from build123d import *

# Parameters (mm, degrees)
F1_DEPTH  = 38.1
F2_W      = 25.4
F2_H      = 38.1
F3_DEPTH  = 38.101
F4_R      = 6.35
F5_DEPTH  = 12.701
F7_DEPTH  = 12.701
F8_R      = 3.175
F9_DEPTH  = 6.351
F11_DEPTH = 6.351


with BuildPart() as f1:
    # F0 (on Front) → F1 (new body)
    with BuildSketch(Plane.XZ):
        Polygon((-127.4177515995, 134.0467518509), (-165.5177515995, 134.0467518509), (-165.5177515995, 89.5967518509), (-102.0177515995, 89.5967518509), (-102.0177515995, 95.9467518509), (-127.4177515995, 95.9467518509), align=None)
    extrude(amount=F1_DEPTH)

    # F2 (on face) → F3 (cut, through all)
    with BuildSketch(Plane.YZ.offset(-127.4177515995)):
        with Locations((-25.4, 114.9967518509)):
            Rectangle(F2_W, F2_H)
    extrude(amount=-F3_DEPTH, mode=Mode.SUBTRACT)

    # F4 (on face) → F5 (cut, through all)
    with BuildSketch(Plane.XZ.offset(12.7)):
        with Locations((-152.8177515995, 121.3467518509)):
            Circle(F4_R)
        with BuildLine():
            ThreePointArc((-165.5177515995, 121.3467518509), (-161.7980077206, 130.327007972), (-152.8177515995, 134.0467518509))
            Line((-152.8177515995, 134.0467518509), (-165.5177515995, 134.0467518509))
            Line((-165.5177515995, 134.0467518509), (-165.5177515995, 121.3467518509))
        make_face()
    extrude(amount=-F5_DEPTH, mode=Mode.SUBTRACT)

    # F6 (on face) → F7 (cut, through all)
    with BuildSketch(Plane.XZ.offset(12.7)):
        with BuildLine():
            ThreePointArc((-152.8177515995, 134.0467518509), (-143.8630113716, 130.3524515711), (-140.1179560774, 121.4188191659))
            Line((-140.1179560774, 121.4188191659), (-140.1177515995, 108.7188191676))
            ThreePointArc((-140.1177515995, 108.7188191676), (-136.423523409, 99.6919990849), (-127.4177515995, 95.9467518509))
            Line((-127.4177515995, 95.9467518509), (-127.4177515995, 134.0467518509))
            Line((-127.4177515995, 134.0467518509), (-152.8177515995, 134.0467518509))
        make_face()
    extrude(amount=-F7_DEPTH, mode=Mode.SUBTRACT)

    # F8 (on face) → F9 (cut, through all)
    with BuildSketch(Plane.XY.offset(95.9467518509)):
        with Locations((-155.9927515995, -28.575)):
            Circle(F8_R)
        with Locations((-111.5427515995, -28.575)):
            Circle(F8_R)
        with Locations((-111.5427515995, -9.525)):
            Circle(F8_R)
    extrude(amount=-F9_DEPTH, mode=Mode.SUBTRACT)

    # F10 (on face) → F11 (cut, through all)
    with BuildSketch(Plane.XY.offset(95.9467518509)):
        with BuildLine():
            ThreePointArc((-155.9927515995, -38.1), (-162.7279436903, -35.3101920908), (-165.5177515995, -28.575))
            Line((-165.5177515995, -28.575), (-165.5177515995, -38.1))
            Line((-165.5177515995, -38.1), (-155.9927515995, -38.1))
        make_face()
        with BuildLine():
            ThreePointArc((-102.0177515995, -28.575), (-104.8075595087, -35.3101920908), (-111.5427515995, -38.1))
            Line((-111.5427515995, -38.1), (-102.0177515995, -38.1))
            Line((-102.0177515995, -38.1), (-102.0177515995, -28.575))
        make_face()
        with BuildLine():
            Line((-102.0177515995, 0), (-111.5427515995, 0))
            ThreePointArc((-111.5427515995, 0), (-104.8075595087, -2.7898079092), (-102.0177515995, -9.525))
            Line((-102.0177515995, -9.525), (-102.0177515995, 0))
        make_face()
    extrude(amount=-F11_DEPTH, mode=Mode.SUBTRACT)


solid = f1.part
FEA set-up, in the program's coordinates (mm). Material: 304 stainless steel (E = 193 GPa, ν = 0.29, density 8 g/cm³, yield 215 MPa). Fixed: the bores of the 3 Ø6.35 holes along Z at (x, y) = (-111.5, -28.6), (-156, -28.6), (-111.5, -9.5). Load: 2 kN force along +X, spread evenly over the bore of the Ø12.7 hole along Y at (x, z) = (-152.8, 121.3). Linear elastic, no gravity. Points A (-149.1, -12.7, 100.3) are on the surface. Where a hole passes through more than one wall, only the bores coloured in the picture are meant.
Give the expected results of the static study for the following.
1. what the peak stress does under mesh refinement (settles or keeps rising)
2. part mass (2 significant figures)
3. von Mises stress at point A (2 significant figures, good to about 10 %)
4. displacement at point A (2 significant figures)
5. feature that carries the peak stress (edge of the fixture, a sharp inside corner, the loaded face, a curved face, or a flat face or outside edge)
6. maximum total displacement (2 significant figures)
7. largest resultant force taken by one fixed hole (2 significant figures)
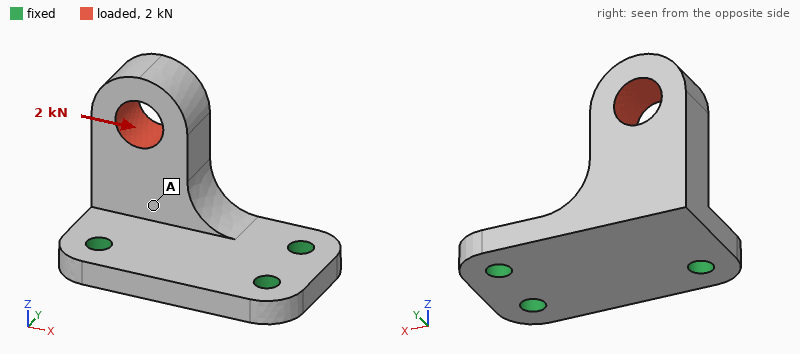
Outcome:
keeps rising
200 g
28 MPa
15 µm
edge of the fixture
80 µm
1.5 kN
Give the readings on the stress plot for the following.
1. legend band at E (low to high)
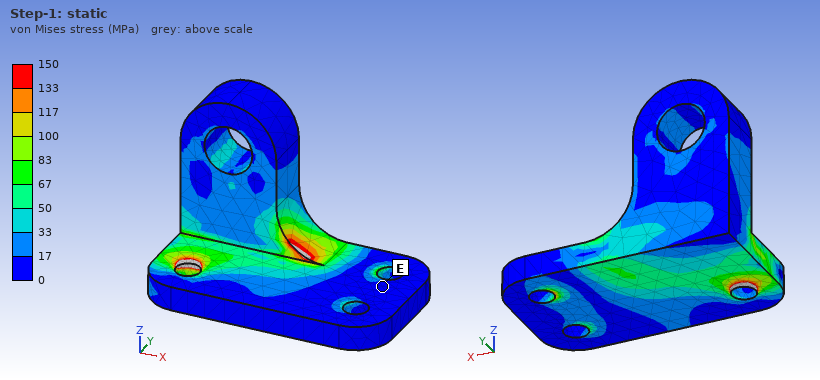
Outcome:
0 to 17 MPa
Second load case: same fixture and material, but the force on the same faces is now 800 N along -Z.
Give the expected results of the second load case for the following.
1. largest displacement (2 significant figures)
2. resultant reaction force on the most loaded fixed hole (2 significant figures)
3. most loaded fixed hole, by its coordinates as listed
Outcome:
36 µm
650 N
(-156, -28.6)
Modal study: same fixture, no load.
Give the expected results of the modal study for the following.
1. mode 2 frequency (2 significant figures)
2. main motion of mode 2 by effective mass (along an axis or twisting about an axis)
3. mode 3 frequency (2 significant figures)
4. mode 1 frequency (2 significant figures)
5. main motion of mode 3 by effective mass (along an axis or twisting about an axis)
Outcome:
4900 Hz
along X
7400 Hz
2300 Hz
along Z
